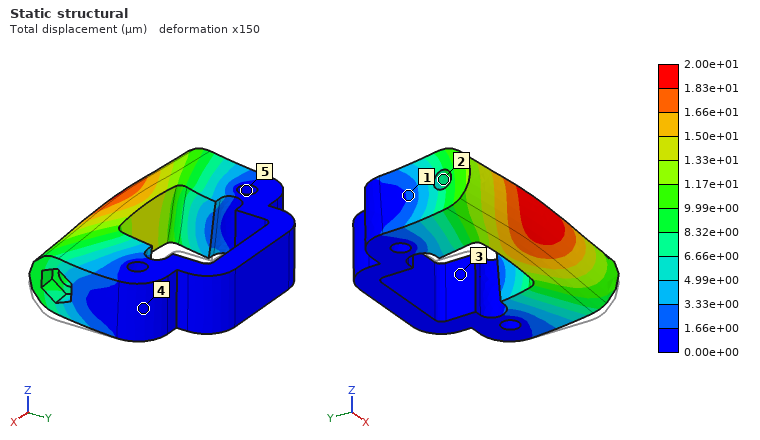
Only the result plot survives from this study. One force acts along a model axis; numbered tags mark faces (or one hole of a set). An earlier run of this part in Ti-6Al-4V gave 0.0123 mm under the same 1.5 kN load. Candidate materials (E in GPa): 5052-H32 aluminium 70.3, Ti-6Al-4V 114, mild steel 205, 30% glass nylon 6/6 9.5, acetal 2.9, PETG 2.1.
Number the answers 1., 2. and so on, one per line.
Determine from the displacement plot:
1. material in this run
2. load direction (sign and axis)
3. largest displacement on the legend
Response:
1. 5052-H32 aluminium
2. +Z
3. 2.00e+01 µm
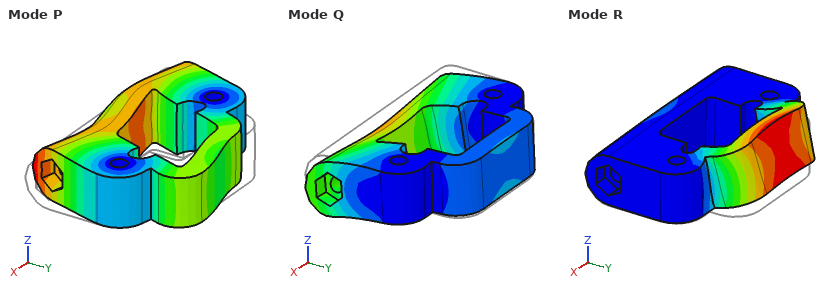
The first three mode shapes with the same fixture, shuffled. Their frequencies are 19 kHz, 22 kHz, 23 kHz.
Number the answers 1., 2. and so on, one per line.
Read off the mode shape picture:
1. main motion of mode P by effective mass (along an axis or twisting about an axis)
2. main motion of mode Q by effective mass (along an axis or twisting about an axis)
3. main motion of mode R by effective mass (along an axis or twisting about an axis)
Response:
1. along X
2. along Z
3. along Z
